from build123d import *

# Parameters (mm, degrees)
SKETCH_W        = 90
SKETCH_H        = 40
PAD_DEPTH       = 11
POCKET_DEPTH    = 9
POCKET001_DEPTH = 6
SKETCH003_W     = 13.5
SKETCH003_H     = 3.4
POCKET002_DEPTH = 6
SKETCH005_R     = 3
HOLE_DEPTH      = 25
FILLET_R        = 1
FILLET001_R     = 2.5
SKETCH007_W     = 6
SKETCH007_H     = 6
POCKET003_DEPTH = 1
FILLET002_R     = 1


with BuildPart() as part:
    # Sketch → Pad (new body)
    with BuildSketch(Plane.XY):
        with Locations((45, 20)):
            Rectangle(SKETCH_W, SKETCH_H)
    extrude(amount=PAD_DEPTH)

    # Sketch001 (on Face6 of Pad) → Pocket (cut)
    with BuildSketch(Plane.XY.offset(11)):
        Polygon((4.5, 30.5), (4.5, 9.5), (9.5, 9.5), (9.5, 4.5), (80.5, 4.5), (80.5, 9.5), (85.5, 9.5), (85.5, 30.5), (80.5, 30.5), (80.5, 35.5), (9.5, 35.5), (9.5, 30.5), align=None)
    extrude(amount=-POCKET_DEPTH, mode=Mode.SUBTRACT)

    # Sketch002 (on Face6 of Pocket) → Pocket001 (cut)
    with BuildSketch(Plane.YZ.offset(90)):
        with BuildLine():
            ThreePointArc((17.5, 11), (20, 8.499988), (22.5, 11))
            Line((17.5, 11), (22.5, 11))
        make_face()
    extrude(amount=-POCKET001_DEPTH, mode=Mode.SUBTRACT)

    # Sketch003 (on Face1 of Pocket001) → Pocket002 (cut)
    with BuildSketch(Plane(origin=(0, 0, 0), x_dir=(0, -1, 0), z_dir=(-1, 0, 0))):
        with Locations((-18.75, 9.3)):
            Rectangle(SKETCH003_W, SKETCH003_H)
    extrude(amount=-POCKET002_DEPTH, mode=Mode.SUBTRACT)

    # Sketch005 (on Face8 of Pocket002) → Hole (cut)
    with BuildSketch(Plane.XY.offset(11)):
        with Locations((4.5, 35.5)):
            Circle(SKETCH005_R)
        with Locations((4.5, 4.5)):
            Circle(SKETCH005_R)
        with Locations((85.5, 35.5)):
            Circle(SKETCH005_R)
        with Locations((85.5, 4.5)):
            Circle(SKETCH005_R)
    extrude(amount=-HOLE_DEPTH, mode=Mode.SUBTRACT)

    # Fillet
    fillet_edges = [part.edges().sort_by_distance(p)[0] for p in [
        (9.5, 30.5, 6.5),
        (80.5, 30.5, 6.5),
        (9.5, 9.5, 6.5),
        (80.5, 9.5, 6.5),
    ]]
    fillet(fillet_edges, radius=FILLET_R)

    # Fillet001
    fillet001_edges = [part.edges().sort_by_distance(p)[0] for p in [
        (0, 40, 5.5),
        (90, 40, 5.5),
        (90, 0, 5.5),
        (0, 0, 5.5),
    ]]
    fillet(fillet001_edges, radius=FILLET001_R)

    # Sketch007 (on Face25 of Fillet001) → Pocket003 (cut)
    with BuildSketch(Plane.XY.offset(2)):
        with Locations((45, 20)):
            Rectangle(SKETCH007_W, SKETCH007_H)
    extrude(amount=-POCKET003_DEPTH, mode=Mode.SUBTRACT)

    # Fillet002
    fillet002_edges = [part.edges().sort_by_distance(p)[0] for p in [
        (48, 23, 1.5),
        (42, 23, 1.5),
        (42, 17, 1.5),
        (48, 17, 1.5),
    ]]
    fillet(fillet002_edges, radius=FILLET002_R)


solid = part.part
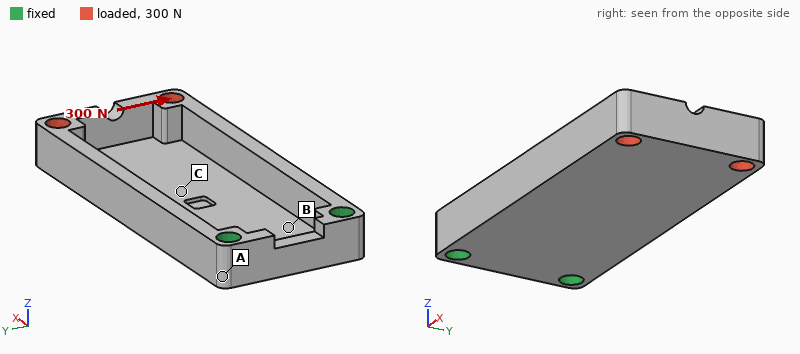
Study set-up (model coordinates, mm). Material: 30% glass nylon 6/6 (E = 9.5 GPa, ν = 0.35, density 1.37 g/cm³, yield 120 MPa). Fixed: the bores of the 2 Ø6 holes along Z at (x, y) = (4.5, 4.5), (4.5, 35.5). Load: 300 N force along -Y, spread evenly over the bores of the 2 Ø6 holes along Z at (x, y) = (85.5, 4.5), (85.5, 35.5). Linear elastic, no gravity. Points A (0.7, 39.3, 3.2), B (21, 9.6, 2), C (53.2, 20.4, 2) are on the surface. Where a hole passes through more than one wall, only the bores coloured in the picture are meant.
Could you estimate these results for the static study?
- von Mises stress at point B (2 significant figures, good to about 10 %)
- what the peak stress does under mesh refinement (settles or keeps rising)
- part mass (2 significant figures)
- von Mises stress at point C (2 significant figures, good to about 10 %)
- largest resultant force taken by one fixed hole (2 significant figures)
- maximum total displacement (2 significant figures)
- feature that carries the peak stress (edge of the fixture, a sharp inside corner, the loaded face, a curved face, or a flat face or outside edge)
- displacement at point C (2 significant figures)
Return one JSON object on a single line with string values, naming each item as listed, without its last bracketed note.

{"von Mises stress at point B": "14 MPa", "what the peak stress does under mesh refinement": "keeps rising", "part mass": "22 g", "von Mises stress at point C": "16 MPa", "largest resultant force taken by one fixed hole": "710 N", "maximum total displacement": "0.97 mm", "feature that carries the peak stress": "edge of the fixture", "displacement at point C": "0.19 mm"}
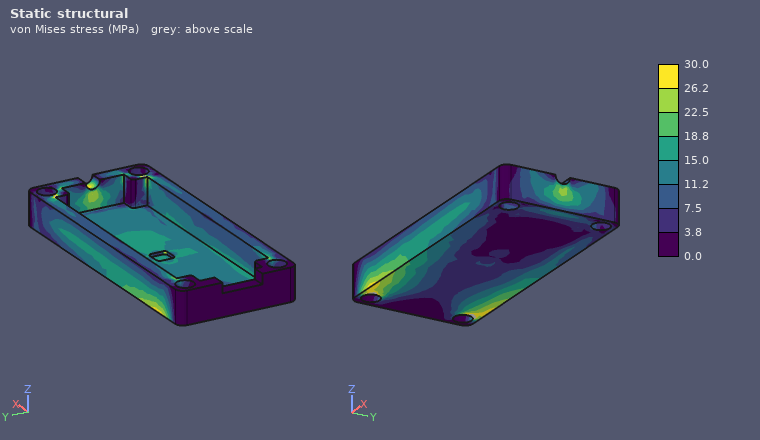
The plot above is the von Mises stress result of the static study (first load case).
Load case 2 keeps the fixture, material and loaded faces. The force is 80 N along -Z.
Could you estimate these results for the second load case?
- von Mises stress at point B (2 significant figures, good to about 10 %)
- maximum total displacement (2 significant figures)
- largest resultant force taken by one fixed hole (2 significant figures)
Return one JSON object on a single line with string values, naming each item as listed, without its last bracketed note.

{"von Mises stress at point B": "4.6 MPa", "maximum total displacement": "0.93 mm", "largest resultant force taken by one fixed hole": "71 N"}
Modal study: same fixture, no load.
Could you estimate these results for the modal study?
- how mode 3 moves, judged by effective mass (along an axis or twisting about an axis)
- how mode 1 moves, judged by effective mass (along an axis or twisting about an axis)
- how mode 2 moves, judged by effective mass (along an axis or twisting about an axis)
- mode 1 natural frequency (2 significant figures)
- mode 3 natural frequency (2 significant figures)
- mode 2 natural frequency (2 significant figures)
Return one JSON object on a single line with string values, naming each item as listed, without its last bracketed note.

{"how mode 3 moves, judged by effective mass": "along Y", "how mode 1 moves, judged by effective mass": "along Z", "how mode 2 moves, judged by effective mass": "along Y", "mode 1 natural frequency": "590 Hz", "mode 3 natural frequency": "2300 Hz", "mode 2 natural frequency": "980 Hz"}
